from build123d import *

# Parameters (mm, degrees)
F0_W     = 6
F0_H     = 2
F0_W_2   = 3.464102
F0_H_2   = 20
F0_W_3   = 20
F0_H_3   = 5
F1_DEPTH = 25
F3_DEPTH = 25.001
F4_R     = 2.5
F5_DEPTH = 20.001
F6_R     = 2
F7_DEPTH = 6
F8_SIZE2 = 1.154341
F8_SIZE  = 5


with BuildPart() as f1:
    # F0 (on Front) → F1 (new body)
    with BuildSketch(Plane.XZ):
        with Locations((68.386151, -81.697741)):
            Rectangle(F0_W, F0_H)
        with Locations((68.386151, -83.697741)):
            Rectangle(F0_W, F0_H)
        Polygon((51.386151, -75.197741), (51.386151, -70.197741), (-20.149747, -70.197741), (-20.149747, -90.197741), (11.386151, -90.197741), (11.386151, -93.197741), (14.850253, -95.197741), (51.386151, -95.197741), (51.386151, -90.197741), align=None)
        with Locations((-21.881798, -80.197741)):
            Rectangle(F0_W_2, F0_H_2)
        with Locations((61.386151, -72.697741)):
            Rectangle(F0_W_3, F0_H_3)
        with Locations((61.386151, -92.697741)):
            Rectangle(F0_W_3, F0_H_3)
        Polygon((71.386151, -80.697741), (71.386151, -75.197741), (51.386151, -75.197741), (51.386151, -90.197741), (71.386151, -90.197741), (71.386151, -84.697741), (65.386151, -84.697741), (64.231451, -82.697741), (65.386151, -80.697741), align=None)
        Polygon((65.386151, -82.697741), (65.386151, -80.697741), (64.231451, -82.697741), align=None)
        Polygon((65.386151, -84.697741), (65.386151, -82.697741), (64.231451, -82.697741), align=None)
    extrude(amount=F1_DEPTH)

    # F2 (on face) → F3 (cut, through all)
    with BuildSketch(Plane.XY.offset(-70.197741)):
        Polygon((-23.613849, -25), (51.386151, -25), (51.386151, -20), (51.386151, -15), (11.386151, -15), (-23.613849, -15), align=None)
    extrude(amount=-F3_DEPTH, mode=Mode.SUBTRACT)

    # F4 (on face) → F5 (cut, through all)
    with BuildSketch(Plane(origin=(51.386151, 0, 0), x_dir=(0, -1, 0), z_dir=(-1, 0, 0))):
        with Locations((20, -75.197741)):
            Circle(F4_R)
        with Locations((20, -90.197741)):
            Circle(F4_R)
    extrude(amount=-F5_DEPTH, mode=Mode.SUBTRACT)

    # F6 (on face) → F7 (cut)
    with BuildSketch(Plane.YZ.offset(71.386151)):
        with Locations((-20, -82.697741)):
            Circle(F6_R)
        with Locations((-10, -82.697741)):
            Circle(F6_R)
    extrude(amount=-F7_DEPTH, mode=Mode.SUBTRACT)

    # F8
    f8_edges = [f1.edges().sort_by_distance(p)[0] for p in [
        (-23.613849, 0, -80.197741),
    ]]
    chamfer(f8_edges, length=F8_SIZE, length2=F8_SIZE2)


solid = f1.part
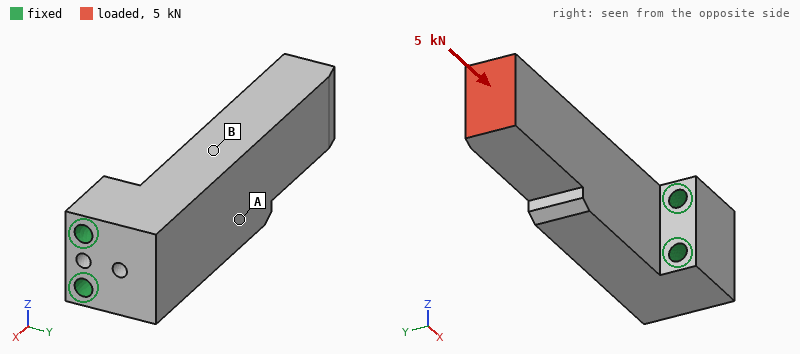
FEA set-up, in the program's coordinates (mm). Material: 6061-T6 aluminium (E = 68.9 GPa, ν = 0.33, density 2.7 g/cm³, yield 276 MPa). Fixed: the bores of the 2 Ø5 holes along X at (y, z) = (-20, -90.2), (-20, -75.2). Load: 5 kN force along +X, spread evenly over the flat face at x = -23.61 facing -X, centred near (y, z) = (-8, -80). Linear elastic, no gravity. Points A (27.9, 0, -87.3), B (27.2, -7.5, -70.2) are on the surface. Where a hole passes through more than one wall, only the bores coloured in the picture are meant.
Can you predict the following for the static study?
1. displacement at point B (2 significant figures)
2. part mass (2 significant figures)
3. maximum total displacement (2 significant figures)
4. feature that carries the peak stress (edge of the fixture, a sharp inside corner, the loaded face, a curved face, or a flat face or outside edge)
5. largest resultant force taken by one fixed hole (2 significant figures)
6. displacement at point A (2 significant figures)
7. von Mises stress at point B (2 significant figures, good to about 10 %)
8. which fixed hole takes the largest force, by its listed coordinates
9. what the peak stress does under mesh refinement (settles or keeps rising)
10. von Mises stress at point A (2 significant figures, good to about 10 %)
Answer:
24 µm
100 g
51 µm
edge of the fixture
3.0 kN
21 µm
21 MPa
(-20, -75.2)
keeps rising
7.9 MPa
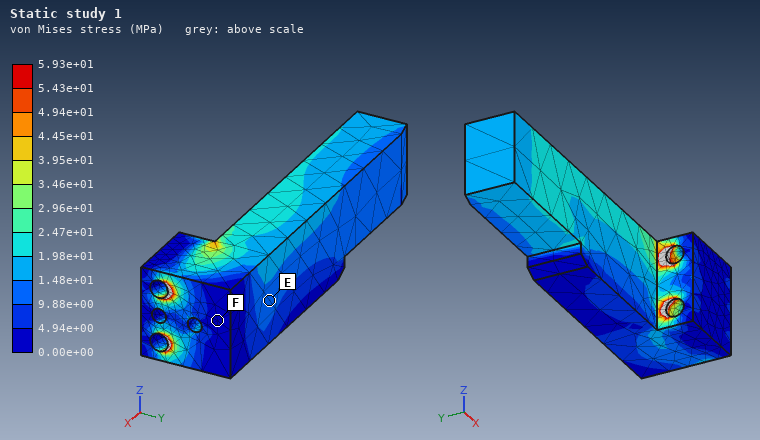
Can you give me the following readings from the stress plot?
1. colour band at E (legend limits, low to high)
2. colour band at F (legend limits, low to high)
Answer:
9.88e+00 to 1.48e+01 MPa
0.00e+00 to 4.94e+00 MPa
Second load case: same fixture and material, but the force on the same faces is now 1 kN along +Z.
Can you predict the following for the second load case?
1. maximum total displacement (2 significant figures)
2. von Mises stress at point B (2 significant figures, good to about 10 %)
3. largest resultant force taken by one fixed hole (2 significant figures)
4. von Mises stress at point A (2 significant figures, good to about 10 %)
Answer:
0.22 mm
34 MPa
3.4 kN
15 MPa
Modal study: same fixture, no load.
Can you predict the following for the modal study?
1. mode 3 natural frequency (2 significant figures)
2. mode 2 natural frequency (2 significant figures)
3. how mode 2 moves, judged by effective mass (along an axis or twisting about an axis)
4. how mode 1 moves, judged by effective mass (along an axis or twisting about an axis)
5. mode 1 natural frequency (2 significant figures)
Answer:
9000 Hz
2600 Hz
along Z
along Y
1800 Hz
